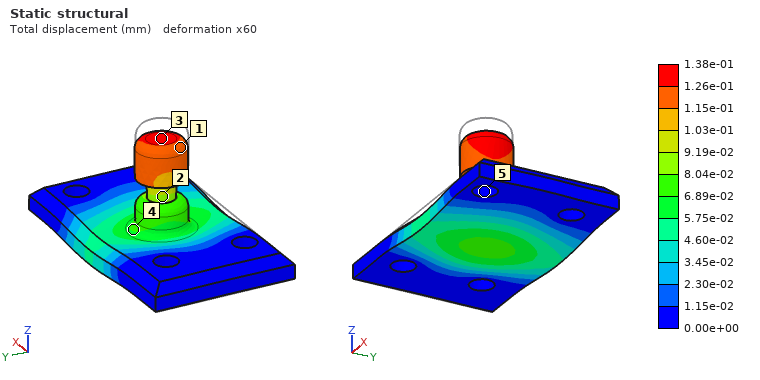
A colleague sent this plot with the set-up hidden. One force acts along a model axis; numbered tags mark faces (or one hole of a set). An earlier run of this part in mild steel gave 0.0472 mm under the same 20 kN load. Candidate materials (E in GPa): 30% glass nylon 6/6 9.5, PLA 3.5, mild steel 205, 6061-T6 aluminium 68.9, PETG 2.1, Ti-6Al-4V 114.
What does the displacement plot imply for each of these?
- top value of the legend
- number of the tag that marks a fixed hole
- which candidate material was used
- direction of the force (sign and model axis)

1.38e-01 mm
5
6061-T6 aluminium
-Z
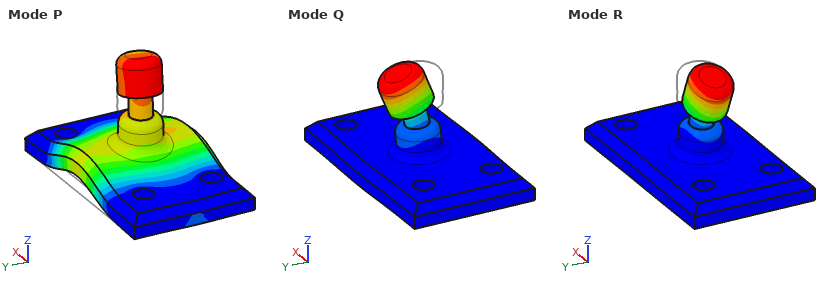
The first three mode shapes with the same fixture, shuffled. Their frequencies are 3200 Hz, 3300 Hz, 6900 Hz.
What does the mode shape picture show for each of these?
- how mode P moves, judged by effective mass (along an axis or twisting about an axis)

along Z
